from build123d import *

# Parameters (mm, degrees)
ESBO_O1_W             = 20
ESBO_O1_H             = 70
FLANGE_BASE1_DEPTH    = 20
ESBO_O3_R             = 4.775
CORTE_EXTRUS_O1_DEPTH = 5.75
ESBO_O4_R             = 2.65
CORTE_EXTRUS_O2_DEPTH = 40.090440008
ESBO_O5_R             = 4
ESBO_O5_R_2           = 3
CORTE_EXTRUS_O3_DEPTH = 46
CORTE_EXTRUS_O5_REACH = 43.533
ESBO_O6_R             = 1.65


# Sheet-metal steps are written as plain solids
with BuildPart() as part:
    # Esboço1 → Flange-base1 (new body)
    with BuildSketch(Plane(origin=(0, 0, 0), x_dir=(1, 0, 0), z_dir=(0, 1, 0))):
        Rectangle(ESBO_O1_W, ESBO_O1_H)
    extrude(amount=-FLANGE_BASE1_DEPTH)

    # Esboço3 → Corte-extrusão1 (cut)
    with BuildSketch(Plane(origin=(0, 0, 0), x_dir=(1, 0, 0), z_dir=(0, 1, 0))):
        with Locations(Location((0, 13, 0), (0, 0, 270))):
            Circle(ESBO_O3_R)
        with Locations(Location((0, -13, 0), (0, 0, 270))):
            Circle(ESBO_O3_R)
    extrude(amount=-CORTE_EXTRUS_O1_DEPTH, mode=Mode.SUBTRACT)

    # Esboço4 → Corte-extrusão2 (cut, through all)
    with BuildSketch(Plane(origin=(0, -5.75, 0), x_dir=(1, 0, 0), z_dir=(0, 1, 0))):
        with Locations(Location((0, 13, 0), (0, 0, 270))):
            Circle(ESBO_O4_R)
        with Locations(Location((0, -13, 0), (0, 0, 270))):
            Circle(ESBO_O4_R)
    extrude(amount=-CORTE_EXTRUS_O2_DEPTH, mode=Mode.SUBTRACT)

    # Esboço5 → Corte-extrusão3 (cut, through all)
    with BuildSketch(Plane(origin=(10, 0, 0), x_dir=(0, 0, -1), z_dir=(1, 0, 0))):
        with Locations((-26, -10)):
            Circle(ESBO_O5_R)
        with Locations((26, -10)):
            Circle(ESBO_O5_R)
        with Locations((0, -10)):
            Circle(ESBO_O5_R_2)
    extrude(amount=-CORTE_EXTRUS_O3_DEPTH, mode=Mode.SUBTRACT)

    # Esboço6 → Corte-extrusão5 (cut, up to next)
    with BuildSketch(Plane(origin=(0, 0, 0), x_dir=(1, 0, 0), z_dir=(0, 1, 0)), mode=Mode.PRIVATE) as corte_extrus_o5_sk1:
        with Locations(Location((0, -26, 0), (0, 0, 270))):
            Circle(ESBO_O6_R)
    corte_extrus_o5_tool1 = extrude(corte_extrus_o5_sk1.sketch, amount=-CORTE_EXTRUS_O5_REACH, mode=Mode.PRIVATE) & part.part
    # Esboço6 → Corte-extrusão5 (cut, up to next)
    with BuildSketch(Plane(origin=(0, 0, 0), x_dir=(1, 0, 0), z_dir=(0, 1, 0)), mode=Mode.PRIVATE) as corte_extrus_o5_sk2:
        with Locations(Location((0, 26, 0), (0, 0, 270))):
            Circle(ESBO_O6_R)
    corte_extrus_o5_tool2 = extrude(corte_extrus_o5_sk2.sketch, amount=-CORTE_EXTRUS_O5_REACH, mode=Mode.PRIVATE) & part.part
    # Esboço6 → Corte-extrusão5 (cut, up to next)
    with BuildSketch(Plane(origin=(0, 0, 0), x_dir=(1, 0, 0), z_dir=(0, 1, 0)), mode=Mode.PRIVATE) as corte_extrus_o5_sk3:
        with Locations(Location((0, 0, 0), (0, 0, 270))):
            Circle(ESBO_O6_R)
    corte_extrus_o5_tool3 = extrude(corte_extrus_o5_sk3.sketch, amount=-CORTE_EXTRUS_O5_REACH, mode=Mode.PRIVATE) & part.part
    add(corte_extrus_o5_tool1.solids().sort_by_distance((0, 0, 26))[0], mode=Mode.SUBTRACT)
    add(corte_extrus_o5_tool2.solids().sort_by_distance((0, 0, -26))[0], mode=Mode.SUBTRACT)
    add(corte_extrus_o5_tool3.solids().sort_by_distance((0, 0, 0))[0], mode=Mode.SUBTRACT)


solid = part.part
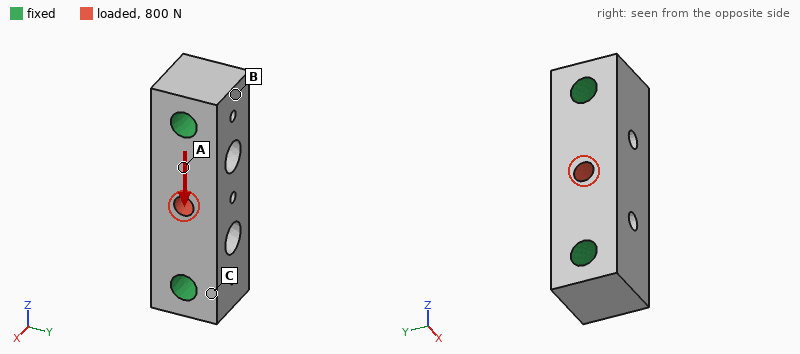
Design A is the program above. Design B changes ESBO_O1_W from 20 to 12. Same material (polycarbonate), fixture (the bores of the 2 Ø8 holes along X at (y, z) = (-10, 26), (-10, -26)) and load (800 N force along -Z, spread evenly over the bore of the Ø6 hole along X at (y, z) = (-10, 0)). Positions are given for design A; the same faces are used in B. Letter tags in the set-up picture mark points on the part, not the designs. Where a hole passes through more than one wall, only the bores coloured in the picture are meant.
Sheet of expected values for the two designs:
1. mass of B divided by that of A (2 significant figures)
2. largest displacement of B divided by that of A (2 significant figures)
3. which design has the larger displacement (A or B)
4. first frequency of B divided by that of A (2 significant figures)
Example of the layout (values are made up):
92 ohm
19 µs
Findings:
0.57
2.0
B
0.74
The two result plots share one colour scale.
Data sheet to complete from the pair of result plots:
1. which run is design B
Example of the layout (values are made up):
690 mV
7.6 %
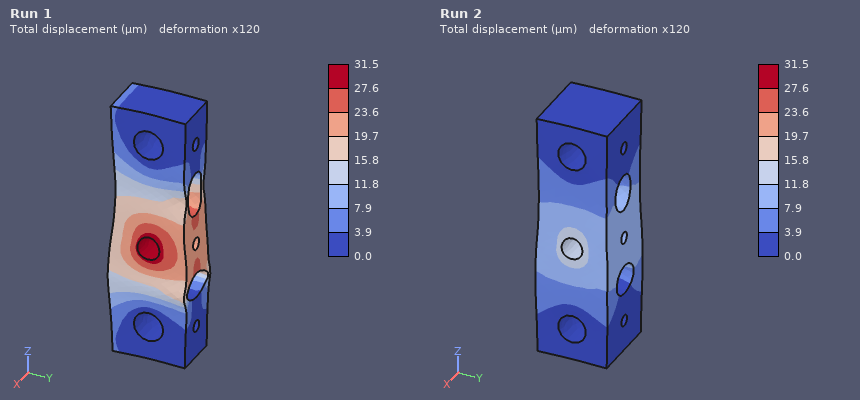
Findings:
Run 1
